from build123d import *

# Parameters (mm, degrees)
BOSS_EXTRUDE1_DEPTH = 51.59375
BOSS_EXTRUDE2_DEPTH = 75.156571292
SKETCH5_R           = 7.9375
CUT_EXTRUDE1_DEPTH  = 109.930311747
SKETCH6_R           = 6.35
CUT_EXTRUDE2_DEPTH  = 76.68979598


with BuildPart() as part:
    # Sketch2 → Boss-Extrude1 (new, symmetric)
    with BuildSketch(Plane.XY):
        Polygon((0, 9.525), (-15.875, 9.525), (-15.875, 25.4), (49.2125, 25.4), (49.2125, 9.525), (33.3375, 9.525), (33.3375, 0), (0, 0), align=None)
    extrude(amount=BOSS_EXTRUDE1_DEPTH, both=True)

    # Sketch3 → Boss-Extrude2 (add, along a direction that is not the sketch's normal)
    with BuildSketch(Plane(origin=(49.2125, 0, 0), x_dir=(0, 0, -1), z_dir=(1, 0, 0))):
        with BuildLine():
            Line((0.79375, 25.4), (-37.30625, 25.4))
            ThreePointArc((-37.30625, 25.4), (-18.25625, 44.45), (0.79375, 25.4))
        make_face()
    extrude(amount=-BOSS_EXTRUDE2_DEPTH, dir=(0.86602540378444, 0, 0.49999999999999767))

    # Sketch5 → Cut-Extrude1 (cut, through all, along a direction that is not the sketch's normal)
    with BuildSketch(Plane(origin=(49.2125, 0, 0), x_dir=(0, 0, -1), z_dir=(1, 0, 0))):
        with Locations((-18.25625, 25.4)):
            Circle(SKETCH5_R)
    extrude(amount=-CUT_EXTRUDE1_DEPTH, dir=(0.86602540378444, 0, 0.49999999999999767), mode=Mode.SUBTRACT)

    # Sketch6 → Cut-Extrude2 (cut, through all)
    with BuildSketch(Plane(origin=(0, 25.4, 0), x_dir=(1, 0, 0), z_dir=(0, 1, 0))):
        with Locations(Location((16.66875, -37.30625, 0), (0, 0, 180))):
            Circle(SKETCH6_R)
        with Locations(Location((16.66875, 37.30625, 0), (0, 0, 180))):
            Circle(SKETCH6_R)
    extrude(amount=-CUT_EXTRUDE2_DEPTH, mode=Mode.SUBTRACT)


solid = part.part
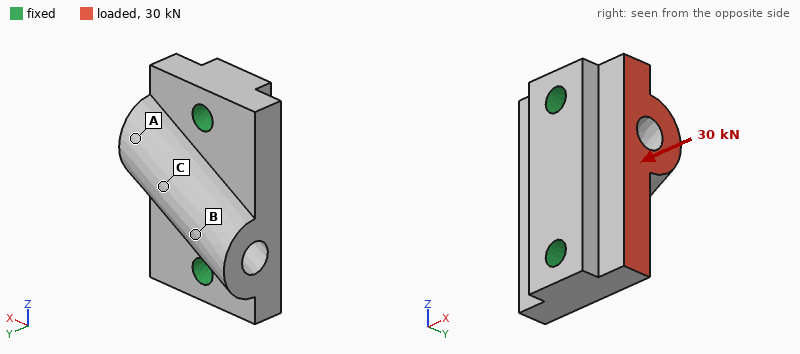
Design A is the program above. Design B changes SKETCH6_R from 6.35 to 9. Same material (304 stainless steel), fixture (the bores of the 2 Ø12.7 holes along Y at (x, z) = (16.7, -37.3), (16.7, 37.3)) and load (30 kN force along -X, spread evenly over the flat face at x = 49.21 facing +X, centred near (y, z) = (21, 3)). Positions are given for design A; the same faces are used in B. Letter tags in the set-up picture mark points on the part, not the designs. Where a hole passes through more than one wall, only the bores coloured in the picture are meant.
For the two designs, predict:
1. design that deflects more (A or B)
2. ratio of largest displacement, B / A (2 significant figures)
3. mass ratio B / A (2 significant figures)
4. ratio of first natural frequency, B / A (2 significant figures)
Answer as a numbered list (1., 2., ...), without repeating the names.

1. A
2. 0.88
3. 0.96
4. 1.1
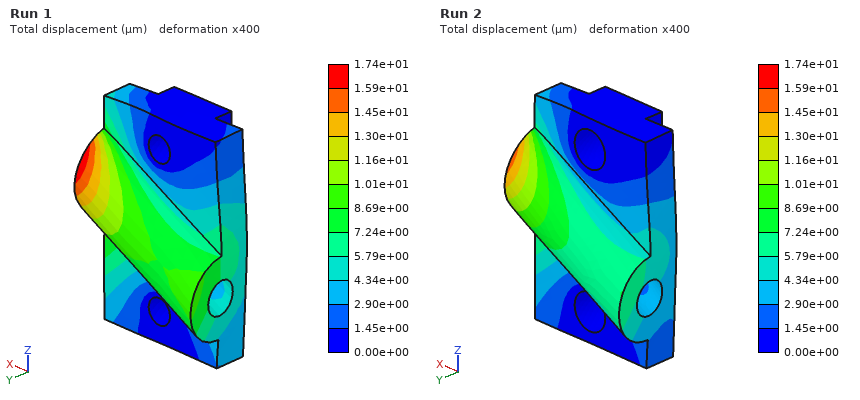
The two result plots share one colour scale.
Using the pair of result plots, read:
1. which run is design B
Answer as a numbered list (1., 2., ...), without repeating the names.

1. Run 2
